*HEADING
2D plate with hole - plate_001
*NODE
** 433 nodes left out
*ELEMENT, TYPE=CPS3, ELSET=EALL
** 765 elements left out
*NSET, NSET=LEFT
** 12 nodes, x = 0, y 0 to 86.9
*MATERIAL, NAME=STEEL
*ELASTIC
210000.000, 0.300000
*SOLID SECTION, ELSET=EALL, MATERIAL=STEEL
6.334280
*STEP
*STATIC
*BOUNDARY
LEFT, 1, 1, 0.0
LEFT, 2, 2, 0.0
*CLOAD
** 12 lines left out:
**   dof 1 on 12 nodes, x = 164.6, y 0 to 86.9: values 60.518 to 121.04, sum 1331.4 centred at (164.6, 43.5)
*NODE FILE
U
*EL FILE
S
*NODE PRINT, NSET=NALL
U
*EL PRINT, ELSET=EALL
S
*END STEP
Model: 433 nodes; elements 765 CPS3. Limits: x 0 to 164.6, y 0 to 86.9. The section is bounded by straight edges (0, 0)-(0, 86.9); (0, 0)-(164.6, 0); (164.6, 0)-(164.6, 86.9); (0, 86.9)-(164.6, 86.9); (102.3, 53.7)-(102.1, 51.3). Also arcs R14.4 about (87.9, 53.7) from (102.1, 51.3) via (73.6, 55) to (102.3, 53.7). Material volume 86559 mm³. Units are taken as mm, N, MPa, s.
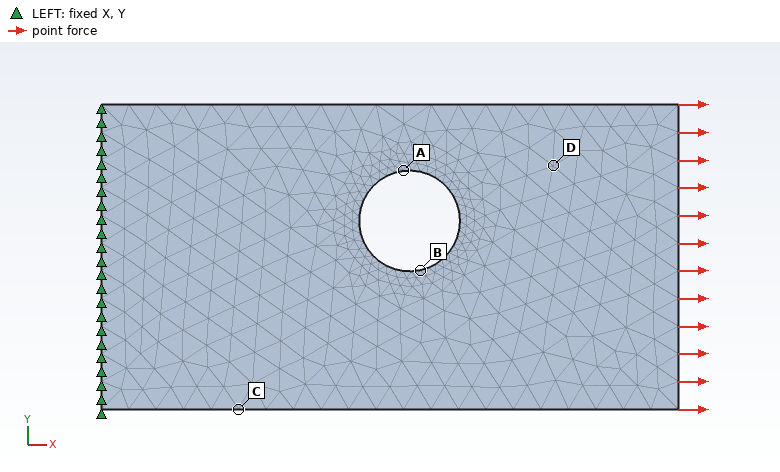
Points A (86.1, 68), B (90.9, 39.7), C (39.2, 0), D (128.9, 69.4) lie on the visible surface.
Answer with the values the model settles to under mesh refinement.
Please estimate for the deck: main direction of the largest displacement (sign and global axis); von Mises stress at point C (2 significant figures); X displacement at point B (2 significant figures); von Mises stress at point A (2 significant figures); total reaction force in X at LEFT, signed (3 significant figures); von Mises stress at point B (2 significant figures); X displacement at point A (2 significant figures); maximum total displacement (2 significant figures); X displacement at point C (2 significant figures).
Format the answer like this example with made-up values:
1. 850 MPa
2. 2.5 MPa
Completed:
1. +X
2. 2.6 MPa
3. 0.0013 mm
4. 9.1 MPa
5. -1330 N
6. 8.1 MPa
7. 0.0011 mm
8. 0.0026 mm
9. 4.8e-04 mm
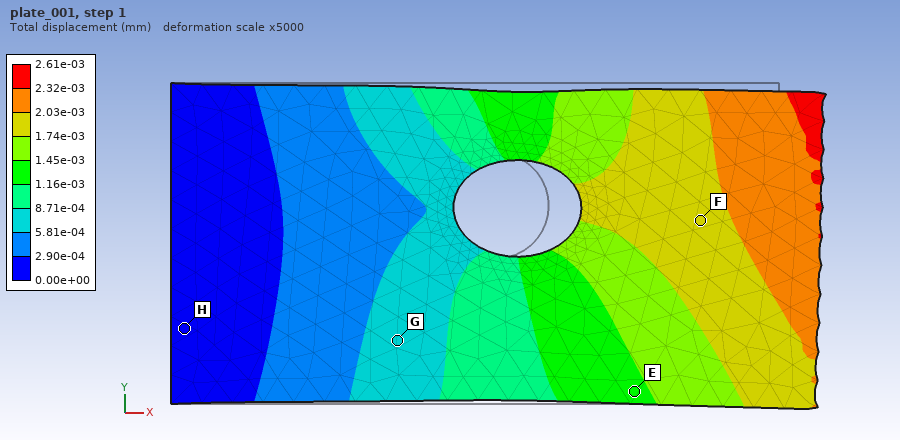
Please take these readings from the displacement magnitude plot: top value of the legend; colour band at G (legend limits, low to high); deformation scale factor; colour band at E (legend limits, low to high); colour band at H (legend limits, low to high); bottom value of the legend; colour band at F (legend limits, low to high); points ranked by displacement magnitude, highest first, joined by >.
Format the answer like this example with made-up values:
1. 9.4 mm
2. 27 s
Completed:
1. 2.61e-03 mm
2. 5.81e-04 to 8.71e-04 mm
3. 5000
4. 1.16e-03 to 1.45e-03 mm
5. 0.00e+00 to 2.90e-04 mm
6. 0.00e+00 mm
7. 1.74e-03 to 2.03e-03 mm
8. F > E > G > H
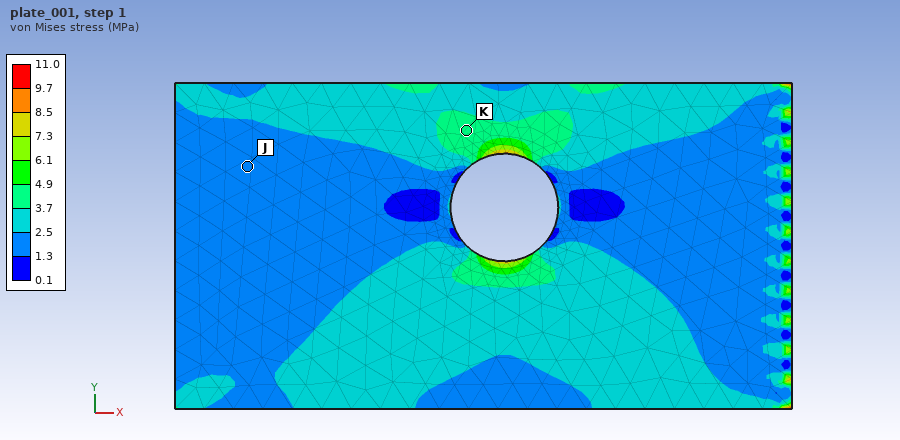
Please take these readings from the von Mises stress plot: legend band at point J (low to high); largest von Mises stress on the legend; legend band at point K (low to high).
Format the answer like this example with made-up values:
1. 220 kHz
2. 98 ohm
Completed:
1. 1.3 to 2.5 MPa
2. 11.0 MPa
3. 3.7 to 4.9 MPa
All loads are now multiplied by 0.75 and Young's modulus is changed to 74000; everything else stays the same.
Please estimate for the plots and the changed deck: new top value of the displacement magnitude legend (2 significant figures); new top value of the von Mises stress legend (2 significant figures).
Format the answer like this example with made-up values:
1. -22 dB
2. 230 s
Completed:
1. 0.0056 mm
2. 8.2 MPa
